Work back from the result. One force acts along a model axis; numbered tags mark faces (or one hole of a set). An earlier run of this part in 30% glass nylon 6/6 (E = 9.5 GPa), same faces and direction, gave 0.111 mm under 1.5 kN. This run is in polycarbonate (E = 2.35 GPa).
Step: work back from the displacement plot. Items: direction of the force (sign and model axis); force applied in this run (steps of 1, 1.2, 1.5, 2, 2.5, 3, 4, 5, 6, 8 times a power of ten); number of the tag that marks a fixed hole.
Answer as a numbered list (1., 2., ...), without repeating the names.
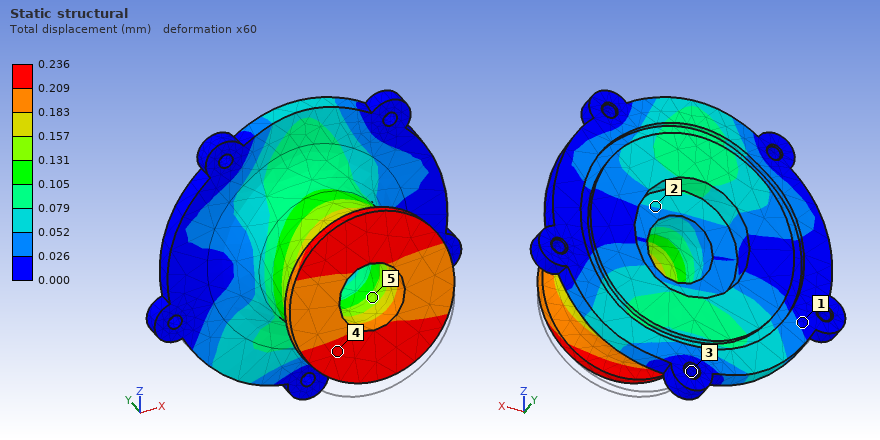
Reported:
1. +Z
2. 800 N
3. 3
